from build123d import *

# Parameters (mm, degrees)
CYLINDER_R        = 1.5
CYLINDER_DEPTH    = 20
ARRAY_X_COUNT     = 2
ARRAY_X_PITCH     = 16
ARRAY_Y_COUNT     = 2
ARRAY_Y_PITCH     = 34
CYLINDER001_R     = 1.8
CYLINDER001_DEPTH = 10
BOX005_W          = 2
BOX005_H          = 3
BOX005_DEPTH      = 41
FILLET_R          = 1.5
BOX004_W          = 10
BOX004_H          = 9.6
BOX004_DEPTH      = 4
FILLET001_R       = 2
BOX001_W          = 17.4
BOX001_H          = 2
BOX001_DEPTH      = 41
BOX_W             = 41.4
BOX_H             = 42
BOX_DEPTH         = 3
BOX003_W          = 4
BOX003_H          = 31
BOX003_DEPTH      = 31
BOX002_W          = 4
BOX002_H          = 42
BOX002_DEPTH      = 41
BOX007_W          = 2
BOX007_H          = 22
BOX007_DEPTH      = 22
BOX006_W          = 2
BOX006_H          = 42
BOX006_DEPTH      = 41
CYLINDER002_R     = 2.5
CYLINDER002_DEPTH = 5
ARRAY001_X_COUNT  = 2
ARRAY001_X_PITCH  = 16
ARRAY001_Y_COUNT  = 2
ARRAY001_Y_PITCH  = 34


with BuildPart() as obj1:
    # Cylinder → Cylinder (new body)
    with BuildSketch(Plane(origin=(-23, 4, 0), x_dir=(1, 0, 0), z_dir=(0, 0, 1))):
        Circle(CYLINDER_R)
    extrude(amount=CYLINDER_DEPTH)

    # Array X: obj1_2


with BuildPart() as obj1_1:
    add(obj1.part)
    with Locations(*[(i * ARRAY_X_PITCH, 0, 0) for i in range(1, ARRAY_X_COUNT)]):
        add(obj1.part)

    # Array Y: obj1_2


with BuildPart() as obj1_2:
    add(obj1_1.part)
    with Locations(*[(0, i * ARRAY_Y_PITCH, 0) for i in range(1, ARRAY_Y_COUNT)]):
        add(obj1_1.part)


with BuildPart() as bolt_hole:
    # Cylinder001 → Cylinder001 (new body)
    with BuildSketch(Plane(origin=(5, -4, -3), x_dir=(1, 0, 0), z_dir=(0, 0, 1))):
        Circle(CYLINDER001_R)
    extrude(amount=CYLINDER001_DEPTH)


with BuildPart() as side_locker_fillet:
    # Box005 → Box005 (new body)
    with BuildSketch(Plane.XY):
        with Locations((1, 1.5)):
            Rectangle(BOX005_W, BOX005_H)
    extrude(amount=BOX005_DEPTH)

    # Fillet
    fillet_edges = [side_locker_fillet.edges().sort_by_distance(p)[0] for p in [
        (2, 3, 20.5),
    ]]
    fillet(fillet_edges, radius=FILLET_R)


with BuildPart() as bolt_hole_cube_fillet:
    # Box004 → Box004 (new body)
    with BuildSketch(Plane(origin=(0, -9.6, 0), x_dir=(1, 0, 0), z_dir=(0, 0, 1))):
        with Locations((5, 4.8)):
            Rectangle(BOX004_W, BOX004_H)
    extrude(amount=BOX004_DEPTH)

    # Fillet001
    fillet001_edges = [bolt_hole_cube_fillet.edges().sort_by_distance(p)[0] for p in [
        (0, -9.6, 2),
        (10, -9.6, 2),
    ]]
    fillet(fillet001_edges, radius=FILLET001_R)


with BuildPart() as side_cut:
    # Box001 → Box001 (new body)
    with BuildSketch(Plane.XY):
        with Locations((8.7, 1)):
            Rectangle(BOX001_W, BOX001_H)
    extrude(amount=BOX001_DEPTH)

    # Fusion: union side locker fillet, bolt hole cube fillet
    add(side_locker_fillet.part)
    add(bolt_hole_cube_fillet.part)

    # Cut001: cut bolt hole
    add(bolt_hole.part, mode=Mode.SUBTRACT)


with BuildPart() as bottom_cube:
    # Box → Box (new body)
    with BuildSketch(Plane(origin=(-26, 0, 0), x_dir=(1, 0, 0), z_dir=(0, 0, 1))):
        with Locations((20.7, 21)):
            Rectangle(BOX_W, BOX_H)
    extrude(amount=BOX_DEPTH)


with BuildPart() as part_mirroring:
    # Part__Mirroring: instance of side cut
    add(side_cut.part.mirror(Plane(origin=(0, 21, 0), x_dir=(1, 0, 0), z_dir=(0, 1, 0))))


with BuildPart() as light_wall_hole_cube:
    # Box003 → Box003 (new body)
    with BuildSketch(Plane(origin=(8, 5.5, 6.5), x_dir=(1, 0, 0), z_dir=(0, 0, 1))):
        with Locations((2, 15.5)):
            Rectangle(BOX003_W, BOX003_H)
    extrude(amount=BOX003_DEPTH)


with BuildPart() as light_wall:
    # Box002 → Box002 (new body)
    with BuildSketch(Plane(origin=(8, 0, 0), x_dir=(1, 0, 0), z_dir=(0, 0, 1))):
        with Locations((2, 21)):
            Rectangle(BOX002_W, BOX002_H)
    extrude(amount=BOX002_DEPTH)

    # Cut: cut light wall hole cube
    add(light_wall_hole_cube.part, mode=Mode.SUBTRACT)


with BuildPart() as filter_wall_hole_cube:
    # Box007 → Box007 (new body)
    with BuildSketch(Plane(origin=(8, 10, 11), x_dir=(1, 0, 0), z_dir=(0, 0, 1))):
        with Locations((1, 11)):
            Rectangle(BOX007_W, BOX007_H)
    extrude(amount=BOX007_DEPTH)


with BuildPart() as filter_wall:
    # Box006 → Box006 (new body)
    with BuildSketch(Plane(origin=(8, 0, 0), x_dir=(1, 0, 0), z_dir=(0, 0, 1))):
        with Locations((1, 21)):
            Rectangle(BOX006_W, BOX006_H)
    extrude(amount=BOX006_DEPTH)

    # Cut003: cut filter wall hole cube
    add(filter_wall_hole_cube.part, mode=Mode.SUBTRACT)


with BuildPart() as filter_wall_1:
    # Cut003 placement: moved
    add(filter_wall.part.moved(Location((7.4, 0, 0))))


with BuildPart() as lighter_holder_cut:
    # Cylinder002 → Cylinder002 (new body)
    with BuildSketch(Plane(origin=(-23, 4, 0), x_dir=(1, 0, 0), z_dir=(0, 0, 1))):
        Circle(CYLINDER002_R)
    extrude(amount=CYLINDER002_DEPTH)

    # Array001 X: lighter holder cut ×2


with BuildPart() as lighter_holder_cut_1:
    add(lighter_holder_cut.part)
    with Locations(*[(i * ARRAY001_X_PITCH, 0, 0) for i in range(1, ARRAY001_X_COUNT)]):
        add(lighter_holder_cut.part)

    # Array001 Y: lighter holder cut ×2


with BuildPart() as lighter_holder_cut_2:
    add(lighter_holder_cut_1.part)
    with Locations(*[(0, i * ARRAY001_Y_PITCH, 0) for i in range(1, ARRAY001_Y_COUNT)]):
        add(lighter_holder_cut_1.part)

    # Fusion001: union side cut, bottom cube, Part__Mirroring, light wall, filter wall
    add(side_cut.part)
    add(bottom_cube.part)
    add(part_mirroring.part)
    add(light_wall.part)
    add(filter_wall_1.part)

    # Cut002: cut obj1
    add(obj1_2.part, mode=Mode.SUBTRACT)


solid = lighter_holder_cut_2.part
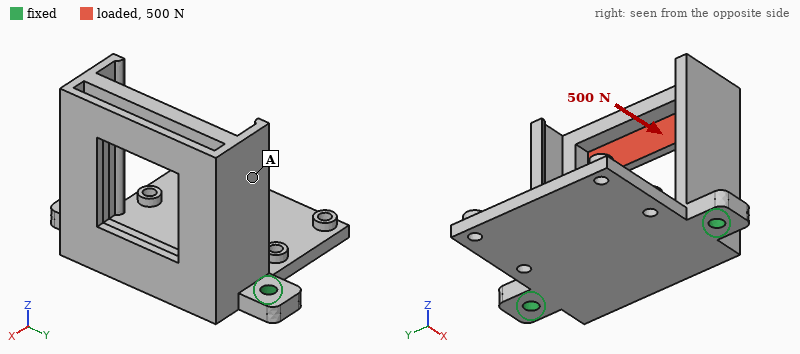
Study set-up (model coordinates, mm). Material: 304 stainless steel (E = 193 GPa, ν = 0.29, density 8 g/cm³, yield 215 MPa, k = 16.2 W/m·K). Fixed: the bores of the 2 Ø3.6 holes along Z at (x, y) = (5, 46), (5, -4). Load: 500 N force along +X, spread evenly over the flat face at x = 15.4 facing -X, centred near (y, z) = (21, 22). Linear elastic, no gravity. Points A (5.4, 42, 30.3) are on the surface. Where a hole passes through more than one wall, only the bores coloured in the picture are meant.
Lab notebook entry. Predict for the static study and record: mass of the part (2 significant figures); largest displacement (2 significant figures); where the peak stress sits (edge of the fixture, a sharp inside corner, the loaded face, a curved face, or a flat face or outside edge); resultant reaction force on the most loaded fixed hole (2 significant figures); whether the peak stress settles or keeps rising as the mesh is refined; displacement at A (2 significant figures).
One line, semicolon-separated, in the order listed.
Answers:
100 g; 0.10 mm; edge of the fixture; 250 N; keeps rising; 0.051 mm
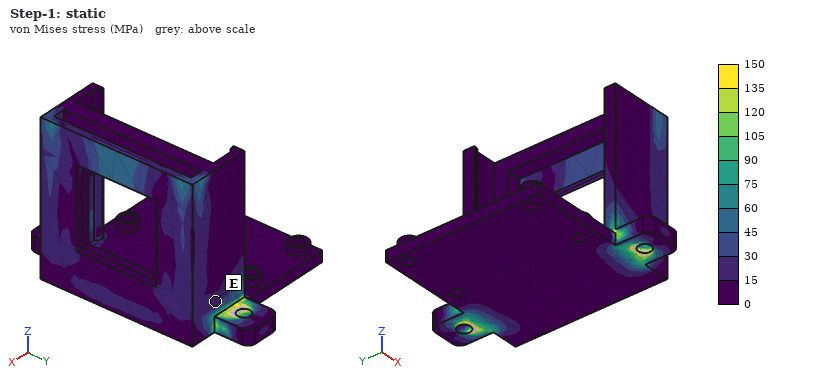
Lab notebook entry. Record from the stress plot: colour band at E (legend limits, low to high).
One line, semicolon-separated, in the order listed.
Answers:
15 to 30 MPa
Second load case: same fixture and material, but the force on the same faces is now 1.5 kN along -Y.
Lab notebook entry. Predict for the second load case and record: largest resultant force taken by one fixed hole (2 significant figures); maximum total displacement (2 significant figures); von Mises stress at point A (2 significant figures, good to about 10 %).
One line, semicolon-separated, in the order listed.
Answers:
1.0 kN; 95 µm; 14 MPa
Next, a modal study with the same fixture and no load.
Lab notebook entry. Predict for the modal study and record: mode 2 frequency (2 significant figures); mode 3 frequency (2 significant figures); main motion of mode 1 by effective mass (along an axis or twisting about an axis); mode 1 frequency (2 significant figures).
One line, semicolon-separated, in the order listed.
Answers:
2700 Hz; 2800 Hz; along X; 1700 Hz
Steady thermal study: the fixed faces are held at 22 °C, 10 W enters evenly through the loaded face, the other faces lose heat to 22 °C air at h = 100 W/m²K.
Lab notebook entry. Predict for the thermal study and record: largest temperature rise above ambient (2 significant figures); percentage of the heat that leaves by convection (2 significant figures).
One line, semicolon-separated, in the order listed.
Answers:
44 K; 89 %
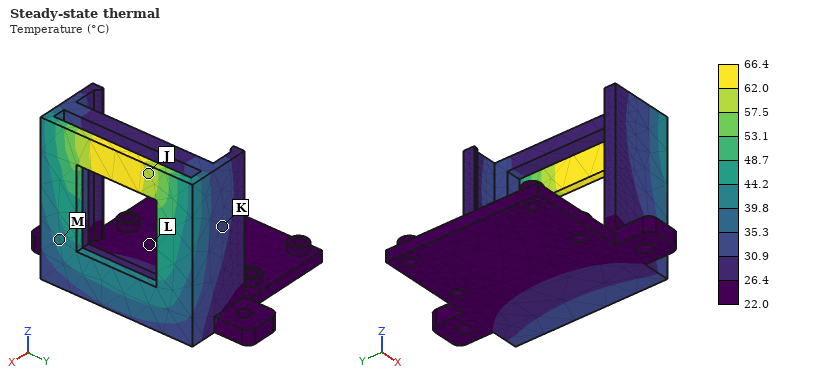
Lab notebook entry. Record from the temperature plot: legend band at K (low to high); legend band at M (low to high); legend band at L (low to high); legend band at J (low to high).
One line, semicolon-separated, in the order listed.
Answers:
30.9 to 35.3 °C; 39.8 to 44.2 °C; 22.0 to 26.4 °C; 57.5 to 62.0 °C
